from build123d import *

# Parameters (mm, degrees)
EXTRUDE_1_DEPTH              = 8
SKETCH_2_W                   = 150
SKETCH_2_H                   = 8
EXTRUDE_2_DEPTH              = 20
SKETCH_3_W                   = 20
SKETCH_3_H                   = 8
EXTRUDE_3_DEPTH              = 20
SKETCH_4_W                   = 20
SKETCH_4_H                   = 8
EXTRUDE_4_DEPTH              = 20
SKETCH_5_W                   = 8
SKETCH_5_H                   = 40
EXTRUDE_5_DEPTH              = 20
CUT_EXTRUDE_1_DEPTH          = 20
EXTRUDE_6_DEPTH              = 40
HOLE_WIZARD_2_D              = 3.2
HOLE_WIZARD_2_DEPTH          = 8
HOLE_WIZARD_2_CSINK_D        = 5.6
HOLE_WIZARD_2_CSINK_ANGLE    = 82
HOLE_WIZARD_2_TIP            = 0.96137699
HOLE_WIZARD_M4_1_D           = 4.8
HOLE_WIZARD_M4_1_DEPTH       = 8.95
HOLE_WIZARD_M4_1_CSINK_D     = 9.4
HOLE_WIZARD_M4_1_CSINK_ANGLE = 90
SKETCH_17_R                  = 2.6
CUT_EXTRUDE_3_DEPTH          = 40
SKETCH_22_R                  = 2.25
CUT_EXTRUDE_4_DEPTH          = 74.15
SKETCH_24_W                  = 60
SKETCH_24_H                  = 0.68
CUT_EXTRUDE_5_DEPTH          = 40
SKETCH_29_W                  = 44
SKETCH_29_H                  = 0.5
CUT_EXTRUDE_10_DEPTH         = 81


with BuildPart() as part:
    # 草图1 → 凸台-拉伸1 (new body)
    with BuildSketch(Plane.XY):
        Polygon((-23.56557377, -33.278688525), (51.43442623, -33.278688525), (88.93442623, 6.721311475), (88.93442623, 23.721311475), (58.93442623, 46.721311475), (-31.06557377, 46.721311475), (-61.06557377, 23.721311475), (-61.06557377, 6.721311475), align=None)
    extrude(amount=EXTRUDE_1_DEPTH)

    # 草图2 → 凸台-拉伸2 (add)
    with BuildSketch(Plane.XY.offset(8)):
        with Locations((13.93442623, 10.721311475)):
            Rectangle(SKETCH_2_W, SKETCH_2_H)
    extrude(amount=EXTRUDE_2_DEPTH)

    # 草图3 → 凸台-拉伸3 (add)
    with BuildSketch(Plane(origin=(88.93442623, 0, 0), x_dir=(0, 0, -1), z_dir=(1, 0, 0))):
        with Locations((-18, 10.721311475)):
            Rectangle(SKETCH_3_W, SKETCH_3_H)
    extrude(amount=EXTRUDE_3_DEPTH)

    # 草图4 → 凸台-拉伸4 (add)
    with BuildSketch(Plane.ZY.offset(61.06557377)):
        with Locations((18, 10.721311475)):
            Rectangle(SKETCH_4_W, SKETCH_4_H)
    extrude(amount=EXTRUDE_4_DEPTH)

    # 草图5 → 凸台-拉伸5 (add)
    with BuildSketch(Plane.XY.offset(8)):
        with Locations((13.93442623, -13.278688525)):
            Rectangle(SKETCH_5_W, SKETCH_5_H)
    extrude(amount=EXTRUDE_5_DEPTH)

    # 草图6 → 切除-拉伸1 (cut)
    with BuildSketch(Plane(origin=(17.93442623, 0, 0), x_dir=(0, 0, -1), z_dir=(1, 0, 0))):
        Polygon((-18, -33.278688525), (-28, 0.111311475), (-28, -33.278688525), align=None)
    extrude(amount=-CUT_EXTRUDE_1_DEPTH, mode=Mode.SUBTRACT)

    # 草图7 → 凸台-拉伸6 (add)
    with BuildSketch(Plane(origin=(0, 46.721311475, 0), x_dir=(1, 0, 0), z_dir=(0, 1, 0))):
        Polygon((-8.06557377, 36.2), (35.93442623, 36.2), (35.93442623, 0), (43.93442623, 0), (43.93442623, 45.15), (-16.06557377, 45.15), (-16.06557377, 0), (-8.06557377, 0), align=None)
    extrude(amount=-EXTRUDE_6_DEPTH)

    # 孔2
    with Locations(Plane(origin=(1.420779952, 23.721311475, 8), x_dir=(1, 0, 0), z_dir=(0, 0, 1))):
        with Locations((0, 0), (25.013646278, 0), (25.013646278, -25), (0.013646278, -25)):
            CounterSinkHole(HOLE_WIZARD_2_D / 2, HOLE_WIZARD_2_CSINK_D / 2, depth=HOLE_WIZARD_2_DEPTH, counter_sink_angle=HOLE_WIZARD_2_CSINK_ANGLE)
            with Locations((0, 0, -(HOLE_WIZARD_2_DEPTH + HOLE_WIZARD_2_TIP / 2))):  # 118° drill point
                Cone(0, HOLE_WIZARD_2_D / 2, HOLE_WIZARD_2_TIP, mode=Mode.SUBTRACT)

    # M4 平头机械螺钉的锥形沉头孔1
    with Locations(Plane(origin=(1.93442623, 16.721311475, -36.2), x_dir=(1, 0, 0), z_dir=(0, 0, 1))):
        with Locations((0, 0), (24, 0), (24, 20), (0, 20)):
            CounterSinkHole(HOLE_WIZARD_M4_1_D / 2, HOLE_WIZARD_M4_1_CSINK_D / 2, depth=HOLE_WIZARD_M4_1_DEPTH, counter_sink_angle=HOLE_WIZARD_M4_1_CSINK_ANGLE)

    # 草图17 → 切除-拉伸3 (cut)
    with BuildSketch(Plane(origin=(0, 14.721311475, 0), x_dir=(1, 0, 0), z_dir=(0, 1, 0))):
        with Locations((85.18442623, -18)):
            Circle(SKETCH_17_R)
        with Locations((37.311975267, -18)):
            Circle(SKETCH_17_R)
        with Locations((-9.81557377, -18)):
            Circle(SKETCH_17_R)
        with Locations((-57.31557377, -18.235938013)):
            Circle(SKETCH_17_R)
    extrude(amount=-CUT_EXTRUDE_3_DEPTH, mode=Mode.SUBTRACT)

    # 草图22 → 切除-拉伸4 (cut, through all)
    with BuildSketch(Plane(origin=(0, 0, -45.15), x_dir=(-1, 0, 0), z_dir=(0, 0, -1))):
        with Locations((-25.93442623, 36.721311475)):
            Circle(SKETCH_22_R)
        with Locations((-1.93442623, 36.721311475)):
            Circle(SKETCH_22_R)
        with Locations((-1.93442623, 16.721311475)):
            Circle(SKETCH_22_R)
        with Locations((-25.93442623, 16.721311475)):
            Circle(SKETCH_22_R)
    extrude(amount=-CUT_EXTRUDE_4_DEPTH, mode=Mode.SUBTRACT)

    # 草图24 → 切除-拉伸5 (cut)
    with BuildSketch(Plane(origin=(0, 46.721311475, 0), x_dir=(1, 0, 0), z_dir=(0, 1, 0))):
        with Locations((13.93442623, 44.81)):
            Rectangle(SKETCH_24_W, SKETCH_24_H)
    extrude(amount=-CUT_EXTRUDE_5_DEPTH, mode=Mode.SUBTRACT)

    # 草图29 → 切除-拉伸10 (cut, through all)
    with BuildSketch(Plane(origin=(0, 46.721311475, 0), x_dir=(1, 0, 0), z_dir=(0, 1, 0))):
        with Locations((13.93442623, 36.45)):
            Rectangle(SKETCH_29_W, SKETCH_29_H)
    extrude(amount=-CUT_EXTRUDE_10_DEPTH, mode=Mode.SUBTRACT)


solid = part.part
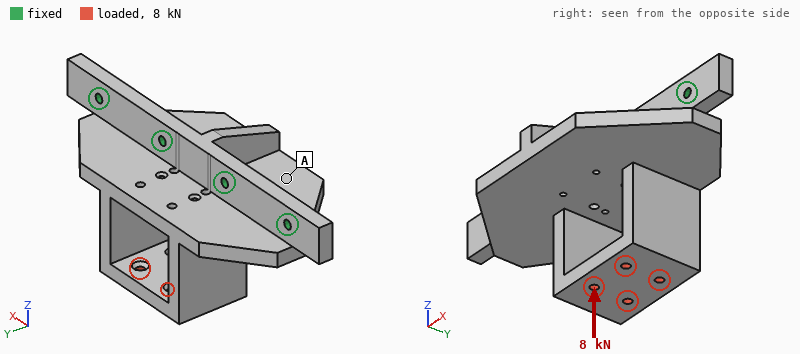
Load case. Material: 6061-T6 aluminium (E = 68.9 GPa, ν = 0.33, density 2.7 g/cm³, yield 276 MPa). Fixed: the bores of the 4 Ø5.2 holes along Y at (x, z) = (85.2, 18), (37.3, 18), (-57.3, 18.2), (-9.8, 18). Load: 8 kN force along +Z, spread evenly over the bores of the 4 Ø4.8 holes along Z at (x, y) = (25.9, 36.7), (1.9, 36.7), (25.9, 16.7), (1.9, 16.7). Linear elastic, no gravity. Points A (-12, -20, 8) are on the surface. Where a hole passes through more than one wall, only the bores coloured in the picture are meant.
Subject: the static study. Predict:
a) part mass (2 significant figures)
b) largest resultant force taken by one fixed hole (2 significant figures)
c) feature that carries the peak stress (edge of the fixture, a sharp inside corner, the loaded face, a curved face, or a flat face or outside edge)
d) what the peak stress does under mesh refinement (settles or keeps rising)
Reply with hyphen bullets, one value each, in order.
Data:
- 420 g
- 3.4 kN
- edge of the fixture
- keeps rising
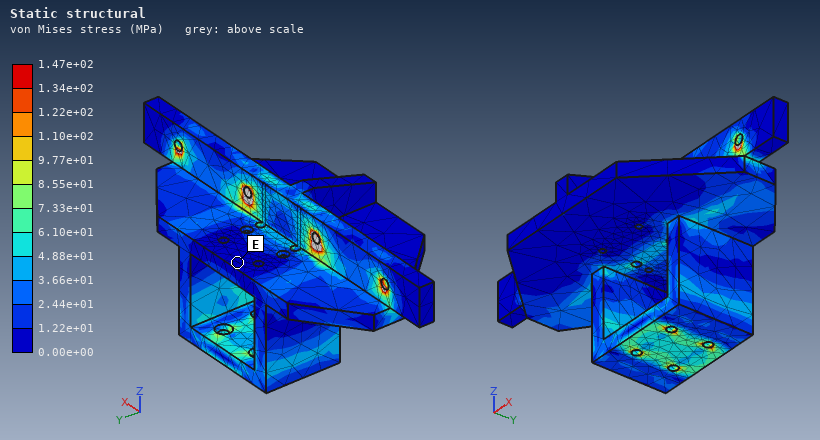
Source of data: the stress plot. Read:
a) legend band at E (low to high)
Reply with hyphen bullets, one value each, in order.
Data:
- 0.00e+00 to 1.22e+01 MPa
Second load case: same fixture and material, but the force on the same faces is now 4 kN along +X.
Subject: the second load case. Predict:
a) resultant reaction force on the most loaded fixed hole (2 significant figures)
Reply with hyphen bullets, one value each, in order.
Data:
- 1.9 kN
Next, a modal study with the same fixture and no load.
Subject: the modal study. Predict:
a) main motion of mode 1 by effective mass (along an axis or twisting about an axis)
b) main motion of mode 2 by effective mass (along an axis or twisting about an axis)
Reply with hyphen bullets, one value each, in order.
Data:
- along Y
- along X
